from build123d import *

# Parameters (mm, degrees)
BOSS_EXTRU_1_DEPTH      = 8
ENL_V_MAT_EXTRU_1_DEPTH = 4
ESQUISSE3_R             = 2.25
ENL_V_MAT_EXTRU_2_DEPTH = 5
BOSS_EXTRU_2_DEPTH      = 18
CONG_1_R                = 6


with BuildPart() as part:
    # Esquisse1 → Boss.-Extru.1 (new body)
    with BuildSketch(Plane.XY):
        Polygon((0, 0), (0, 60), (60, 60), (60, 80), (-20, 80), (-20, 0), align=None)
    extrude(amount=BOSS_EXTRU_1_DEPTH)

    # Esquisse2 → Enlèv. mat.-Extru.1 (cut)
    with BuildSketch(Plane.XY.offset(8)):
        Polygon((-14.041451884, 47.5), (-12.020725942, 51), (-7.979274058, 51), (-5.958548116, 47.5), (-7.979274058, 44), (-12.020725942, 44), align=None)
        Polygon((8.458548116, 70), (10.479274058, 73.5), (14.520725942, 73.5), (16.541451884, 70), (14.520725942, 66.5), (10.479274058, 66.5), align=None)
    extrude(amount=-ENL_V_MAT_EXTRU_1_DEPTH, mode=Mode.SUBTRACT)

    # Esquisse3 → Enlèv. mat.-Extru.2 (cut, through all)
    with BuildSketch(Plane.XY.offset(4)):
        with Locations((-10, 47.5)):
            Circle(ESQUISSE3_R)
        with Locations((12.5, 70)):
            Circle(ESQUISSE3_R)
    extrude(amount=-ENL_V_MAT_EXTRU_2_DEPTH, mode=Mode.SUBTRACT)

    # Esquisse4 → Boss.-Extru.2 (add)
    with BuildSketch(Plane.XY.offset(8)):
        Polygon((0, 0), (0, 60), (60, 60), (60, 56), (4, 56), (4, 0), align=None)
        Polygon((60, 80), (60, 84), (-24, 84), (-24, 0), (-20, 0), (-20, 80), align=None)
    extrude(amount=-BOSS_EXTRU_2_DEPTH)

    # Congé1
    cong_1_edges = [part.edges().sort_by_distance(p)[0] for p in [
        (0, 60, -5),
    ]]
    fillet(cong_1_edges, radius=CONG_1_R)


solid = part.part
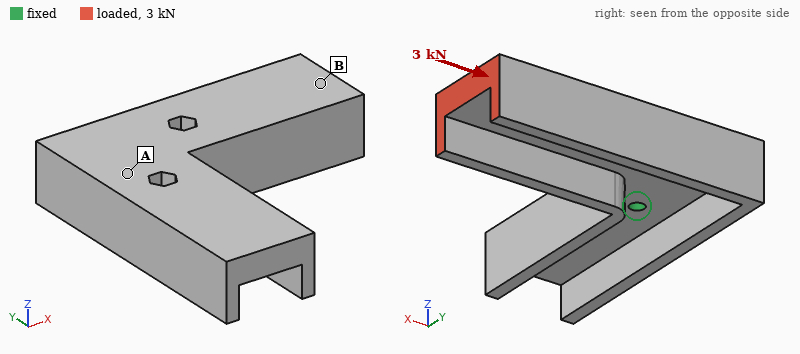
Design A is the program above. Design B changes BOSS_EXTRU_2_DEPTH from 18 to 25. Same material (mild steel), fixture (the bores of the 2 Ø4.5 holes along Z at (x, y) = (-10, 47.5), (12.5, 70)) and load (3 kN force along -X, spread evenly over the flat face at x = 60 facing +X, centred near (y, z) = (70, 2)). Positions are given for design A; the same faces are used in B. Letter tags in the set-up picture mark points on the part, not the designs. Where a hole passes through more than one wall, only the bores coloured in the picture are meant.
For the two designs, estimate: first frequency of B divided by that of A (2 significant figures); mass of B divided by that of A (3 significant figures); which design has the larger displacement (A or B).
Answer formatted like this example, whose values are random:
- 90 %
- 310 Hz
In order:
- 0.90
- 1.19
- B
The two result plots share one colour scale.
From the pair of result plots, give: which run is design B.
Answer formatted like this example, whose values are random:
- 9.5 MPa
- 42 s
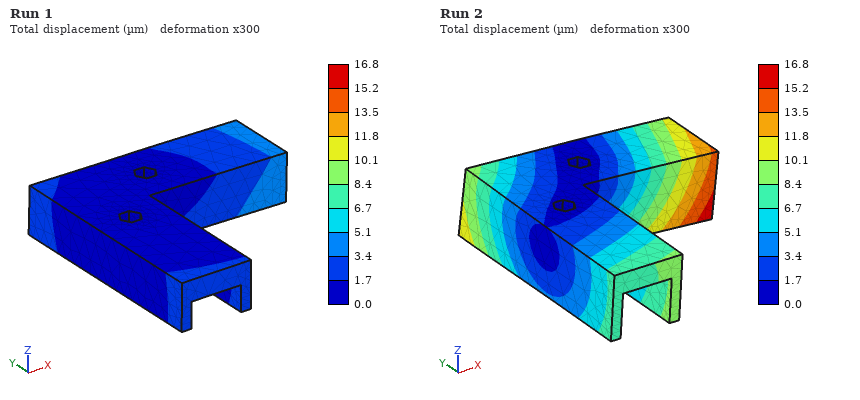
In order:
- Run 2
